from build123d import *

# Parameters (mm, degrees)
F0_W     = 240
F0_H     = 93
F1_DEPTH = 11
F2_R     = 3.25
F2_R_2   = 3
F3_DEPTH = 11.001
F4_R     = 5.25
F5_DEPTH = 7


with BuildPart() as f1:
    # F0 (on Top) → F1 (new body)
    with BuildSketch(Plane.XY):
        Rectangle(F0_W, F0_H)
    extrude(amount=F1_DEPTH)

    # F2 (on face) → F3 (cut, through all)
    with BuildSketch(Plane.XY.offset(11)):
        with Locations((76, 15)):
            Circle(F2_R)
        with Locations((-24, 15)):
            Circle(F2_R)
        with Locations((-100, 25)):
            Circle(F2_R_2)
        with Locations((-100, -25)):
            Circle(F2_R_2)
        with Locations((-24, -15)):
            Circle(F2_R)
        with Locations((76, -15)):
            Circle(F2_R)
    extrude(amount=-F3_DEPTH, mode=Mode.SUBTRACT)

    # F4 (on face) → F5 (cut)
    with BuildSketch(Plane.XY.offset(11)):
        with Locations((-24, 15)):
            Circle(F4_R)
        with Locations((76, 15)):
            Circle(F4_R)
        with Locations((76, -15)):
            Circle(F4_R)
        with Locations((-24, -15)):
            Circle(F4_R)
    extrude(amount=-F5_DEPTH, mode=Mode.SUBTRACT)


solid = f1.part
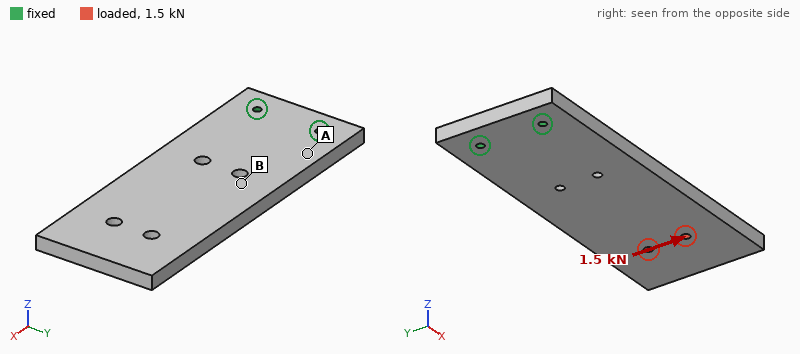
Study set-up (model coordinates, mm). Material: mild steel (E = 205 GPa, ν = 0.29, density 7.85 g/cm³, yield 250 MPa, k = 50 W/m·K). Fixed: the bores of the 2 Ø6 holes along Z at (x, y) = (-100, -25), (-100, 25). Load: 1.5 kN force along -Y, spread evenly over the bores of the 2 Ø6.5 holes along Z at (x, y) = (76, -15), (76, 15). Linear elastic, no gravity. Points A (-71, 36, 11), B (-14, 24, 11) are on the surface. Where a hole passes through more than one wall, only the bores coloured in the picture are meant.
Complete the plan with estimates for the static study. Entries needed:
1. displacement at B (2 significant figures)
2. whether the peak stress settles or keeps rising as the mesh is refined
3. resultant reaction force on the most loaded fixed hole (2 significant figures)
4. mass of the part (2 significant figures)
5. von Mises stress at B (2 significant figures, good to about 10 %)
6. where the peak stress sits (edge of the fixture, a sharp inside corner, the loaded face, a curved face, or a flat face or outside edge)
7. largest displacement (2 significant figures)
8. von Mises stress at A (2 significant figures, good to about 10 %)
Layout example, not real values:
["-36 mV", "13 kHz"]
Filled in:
["11 µm", "keeps rising", "5.1 kN", "1.9 kg", "5.1 MPa", "edge of the fixture", "42 µm", "12 MPa"]
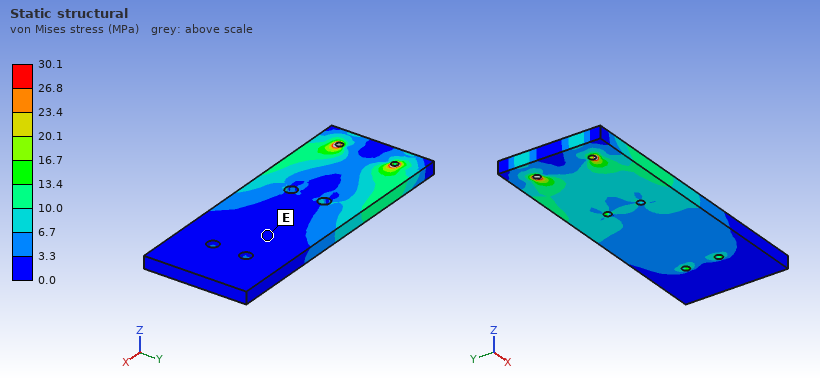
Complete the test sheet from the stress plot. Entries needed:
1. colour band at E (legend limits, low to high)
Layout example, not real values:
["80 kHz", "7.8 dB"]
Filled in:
["0.0 to 3.3 MPa"]
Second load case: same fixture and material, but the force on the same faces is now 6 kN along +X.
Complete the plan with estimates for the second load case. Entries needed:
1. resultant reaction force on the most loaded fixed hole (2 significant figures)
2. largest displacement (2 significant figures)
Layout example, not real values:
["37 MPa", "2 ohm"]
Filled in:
["3.0 kN", "0.24 mm"]
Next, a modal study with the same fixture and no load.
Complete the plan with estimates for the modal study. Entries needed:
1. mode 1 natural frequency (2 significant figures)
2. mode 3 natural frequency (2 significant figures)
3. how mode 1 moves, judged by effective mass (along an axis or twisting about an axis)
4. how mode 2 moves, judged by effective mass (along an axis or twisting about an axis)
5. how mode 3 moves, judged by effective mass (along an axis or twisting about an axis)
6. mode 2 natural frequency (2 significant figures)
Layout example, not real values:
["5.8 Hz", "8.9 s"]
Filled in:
["180 Hz", "1100 Hz", "along Z", "twisting about X", "along Z", "880 Hz"]
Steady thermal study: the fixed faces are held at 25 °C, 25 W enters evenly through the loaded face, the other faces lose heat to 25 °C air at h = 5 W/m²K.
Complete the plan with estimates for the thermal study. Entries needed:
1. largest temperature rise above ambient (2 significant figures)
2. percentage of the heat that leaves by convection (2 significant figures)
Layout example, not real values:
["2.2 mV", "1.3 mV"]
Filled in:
["75 K", "37 %"]
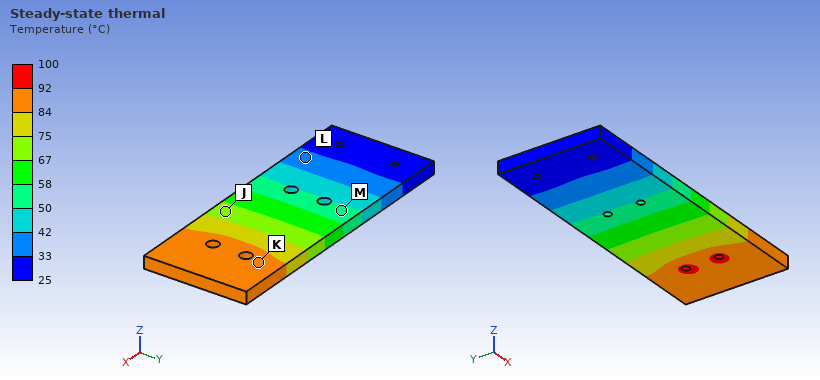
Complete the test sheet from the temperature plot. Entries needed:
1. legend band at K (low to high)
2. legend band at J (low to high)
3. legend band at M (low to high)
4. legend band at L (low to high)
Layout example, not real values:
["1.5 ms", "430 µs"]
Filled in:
["84 to 92 °C", "67 to 75 °C", "50 to 58 °C", "33 to 42 °C"]
